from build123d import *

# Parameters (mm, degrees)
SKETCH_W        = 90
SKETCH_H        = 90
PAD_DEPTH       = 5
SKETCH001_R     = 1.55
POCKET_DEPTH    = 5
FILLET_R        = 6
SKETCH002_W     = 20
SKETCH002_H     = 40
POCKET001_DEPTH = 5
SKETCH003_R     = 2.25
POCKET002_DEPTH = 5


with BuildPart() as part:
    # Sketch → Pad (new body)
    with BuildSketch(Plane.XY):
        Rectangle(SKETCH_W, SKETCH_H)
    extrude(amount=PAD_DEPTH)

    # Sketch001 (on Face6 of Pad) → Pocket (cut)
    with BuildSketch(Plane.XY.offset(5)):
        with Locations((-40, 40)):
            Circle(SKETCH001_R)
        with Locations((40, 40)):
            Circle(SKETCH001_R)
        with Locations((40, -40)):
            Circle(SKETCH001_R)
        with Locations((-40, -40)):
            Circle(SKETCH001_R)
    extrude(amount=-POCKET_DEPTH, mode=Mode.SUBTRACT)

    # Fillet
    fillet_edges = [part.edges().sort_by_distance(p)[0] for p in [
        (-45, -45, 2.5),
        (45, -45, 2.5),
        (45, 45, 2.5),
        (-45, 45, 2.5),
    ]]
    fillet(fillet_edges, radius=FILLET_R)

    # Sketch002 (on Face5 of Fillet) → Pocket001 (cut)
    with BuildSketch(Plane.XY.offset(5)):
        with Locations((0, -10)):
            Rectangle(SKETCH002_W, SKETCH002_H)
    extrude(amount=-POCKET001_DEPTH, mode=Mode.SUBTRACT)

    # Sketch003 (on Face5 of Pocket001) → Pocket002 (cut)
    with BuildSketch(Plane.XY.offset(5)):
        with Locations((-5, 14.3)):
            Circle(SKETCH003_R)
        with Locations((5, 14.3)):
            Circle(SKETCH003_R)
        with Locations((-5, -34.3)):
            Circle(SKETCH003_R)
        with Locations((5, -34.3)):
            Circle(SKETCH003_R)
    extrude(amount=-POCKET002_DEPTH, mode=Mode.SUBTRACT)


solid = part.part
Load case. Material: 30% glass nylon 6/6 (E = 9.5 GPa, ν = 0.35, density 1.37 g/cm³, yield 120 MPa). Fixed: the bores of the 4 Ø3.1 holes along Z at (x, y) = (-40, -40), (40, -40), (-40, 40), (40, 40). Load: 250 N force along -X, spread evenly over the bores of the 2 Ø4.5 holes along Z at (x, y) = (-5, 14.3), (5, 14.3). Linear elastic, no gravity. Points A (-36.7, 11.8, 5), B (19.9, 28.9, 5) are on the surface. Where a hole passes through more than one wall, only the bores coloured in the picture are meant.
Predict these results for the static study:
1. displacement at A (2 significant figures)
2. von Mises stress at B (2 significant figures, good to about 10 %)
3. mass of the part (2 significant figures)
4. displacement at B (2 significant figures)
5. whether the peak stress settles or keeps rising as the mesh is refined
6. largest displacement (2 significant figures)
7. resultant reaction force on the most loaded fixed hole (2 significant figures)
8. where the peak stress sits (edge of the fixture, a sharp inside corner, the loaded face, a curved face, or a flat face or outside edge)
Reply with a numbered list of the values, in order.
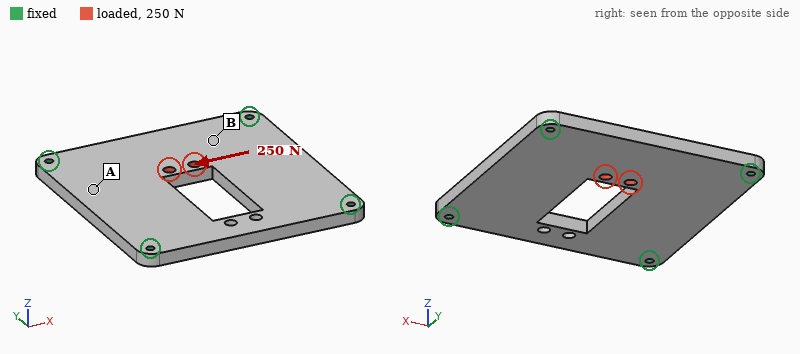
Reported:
1. 4.7 µm
2. 1.1 MPa
3. 49 g
4. 3.7 µm
5. keeps rising
6. 8.9 µm
7. 110 N
8. edge of the fixture
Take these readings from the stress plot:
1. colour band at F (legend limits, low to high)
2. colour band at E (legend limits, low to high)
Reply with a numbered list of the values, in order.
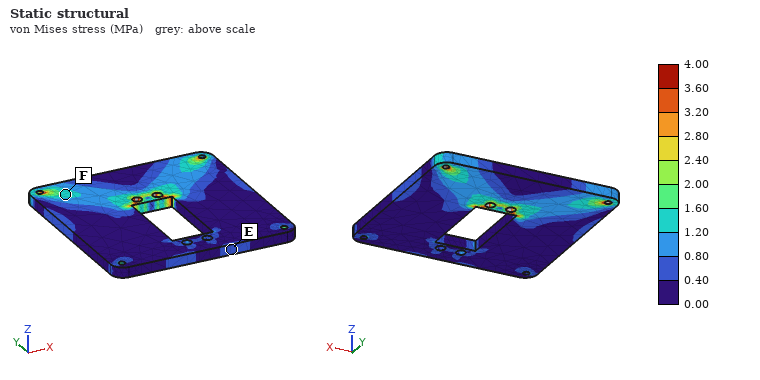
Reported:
1. 1.20 to 1.60 MPa
2. 0.40 to 0.80 MPa
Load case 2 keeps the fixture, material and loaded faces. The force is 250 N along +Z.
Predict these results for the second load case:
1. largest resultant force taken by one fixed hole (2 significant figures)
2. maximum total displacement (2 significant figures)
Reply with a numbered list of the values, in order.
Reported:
1. 88 N
2. 0.42 mm
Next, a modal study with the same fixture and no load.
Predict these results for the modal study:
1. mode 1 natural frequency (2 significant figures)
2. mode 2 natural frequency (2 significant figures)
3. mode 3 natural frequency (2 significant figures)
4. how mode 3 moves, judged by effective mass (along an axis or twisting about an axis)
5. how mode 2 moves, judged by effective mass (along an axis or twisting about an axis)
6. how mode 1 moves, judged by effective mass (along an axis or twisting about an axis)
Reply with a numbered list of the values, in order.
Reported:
1. 1200 Hz
2. 2000 Hz
3. 2200 Hz
4. twisting about X
5. twisting about Y
6. along Z
